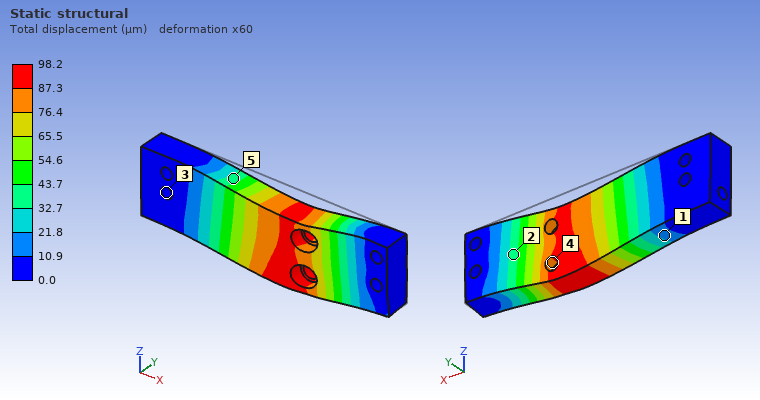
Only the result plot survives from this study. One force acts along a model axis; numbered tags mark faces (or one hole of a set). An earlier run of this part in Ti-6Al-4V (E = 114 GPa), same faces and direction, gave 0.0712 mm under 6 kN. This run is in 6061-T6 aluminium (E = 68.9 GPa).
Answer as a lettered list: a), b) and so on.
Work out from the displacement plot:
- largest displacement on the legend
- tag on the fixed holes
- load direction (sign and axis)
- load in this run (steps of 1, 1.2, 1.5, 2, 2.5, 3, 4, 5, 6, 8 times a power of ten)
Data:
a) 98.2 µm
b) 3
c) -Y
d) 5 kN
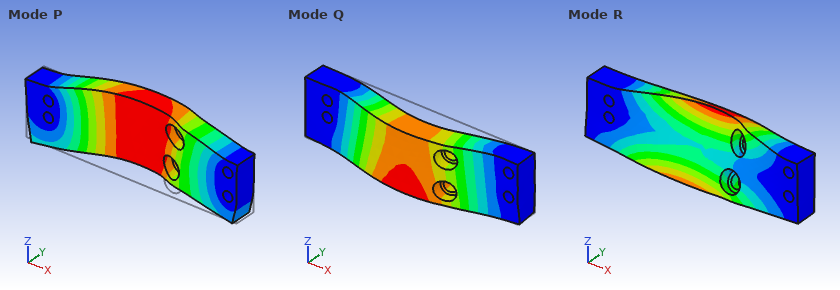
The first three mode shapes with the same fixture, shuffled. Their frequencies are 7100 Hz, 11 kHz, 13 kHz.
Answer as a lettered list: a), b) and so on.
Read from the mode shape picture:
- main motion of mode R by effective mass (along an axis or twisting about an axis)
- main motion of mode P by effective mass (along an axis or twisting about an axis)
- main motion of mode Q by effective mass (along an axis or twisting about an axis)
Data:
a) twisting about X
b) along Z
c) along Y
